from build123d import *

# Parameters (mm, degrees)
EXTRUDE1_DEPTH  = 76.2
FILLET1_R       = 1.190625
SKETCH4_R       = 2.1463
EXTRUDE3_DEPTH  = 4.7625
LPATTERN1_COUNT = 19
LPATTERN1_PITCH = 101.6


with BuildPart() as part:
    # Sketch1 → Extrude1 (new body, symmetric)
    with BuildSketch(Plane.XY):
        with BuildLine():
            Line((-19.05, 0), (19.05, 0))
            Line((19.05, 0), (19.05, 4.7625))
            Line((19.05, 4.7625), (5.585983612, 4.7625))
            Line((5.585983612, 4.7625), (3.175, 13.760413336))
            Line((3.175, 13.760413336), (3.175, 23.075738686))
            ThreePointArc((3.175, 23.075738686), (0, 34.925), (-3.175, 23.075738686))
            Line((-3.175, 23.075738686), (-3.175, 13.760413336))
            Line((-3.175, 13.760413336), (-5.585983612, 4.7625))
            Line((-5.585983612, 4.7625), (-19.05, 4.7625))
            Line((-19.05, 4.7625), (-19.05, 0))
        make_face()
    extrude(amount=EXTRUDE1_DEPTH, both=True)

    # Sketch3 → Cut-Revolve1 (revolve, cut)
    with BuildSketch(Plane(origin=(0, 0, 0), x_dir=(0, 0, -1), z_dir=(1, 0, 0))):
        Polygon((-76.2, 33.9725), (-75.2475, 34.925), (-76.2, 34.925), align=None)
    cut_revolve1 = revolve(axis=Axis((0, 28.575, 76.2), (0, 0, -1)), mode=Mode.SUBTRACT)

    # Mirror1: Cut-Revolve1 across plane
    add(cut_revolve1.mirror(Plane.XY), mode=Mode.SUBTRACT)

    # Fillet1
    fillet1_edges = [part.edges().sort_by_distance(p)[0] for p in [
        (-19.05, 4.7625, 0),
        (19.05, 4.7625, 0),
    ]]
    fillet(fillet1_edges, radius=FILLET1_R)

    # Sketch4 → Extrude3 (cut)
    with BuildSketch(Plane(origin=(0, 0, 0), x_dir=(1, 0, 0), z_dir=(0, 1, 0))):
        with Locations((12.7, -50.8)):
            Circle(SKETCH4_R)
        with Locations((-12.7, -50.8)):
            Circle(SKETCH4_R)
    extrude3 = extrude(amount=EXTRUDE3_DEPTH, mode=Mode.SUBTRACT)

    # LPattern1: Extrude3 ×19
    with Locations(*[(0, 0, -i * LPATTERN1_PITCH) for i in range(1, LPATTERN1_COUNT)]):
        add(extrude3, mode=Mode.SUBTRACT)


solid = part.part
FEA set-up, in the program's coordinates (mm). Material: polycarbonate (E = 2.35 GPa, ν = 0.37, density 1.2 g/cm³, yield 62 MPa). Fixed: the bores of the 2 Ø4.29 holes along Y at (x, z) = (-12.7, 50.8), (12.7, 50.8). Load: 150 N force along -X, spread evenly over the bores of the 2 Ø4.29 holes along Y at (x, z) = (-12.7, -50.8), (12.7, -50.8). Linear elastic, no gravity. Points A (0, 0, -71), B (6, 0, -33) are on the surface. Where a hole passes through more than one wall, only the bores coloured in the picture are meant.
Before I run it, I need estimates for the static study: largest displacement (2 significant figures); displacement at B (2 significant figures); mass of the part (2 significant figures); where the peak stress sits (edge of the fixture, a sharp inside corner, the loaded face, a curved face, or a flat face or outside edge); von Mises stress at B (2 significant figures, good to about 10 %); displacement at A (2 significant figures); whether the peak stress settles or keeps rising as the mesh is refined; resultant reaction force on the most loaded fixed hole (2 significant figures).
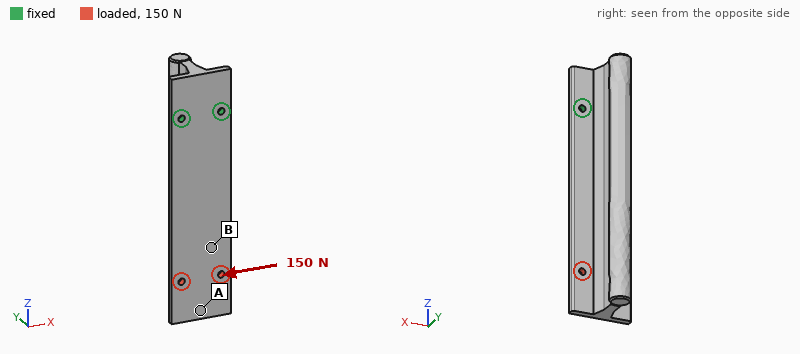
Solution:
1.5 mm
0.83 mm
80 g
edge of the fixture
2.3 MPa
1.4 mm
keeps rising
570 N
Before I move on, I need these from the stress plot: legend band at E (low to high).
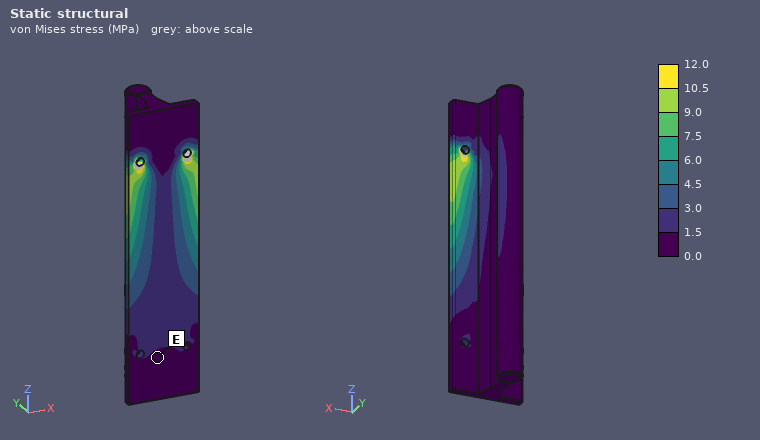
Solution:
0.0 to 1.5 MPa
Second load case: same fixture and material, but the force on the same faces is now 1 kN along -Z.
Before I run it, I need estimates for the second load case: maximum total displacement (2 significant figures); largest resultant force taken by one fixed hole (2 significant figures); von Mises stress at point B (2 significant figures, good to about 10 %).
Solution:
0.57 mm
500 N
4.5 MPa
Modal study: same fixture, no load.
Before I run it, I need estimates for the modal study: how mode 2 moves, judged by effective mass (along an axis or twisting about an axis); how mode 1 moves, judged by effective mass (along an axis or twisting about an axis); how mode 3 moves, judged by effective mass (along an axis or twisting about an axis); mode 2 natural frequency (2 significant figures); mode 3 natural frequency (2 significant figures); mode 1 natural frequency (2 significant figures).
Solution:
along X
along Y
twisting about Z
290 Hz
550 Hz
120 Hz
